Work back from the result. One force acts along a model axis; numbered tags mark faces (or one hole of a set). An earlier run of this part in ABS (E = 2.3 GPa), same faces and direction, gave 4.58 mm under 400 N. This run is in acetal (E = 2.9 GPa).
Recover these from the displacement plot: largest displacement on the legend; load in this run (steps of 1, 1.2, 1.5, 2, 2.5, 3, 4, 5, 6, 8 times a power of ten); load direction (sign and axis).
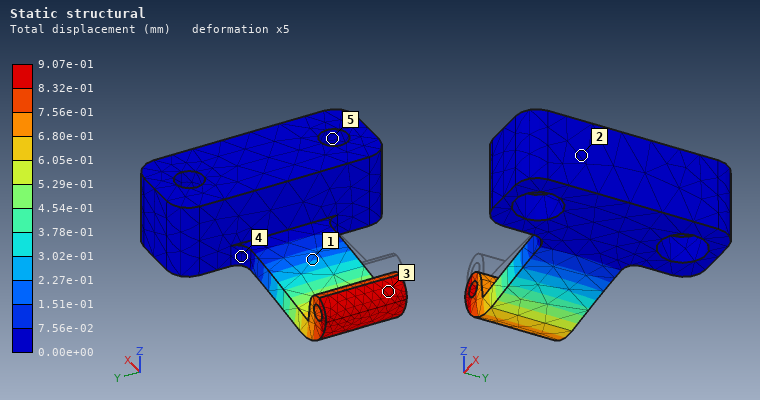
9.07e-01 mm
100 N
-Z
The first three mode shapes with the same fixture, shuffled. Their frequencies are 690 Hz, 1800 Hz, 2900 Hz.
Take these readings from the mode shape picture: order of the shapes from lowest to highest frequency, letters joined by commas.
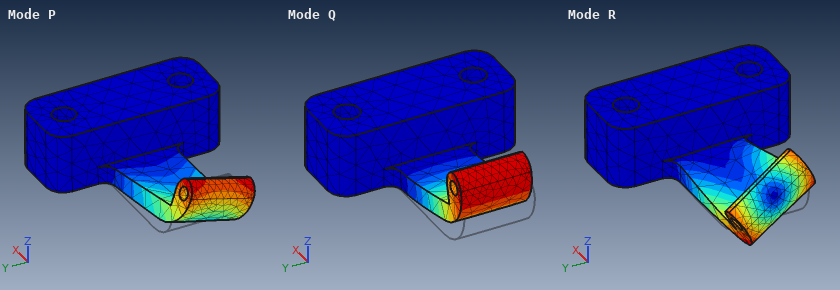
Q, P, R
